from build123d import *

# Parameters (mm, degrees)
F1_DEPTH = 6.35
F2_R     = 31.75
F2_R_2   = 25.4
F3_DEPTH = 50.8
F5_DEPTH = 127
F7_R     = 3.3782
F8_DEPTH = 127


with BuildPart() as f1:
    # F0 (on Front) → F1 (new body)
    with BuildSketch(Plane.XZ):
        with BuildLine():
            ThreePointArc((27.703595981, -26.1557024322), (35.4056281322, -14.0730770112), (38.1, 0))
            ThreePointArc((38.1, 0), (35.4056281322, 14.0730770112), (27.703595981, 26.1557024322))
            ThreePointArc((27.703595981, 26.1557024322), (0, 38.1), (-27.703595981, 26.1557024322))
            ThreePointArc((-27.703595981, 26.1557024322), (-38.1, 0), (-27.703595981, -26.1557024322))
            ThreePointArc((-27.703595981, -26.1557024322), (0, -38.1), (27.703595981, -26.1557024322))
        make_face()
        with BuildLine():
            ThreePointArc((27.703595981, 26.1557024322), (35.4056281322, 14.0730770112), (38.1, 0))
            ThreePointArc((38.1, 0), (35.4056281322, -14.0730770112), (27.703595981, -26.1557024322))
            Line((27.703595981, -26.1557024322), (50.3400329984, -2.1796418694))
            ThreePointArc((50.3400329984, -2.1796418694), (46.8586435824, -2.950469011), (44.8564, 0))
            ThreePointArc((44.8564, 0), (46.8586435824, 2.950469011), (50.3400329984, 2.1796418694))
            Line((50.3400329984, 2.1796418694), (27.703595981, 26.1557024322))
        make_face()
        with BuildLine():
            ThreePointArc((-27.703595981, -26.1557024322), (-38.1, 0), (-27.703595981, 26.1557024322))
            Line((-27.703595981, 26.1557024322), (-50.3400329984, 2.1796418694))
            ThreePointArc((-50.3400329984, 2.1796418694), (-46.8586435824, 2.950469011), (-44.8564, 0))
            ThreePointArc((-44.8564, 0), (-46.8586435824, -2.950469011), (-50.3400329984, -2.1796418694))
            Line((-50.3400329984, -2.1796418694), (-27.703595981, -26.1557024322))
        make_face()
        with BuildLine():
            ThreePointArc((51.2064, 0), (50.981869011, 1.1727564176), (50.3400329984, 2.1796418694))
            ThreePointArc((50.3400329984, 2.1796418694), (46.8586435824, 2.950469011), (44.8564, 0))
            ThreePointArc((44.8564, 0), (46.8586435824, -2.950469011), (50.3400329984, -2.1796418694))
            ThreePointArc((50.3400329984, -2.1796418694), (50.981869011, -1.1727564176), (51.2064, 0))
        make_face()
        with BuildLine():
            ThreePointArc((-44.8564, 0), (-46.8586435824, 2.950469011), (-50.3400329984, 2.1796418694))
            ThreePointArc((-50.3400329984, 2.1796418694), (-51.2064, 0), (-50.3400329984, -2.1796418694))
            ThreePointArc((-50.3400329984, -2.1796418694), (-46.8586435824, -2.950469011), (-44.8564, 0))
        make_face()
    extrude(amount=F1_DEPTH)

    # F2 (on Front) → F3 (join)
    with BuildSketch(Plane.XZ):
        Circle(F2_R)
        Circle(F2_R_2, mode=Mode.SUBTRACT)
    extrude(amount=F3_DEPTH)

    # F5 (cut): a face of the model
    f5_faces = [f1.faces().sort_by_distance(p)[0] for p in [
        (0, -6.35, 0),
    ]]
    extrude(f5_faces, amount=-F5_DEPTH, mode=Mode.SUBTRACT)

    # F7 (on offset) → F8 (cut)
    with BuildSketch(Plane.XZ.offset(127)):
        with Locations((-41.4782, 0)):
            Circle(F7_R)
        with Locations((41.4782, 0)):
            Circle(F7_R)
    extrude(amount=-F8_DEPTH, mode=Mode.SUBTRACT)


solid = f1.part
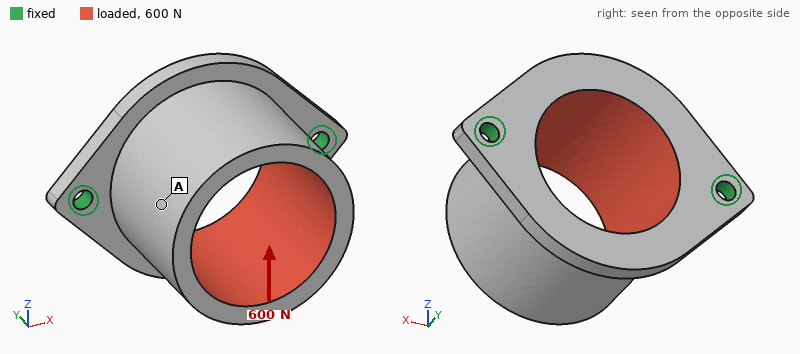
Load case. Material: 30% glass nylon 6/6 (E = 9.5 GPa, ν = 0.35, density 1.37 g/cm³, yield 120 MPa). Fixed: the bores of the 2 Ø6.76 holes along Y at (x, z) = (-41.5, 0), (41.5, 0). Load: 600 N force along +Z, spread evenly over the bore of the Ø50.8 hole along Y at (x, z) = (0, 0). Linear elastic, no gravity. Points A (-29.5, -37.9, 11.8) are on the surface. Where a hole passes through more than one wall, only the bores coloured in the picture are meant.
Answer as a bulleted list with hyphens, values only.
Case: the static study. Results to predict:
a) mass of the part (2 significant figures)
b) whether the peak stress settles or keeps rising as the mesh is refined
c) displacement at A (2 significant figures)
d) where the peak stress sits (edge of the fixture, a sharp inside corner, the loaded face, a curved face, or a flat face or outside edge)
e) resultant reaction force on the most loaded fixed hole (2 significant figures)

- 96 g
- keeps rising
- 0.32 mm
- edge of the fixture
- 300 N
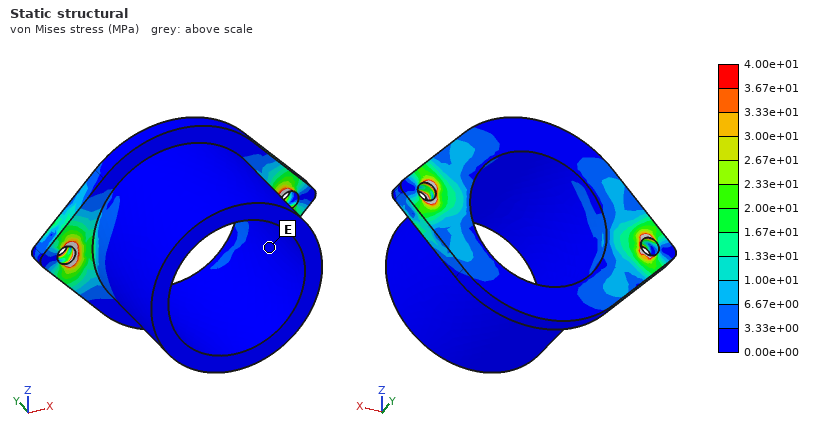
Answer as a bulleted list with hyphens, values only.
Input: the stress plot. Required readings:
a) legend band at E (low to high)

- 0.00e+00 to 3.33e+00 MPa
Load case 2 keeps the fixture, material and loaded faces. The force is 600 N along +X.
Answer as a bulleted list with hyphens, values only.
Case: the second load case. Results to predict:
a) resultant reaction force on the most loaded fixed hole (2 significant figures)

- 350 N
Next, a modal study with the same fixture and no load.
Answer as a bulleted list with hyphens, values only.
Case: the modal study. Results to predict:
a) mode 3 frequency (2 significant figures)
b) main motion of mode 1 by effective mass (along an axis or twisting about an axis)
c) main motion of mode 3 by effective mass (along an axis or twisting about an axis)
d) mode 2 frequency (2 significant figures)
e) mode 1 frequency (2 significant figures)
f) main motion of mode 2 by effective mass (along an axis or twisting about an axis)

- 2800 Hz
- along Z
- along X
- 2100 Hz
- 640 Hz
- along Y
